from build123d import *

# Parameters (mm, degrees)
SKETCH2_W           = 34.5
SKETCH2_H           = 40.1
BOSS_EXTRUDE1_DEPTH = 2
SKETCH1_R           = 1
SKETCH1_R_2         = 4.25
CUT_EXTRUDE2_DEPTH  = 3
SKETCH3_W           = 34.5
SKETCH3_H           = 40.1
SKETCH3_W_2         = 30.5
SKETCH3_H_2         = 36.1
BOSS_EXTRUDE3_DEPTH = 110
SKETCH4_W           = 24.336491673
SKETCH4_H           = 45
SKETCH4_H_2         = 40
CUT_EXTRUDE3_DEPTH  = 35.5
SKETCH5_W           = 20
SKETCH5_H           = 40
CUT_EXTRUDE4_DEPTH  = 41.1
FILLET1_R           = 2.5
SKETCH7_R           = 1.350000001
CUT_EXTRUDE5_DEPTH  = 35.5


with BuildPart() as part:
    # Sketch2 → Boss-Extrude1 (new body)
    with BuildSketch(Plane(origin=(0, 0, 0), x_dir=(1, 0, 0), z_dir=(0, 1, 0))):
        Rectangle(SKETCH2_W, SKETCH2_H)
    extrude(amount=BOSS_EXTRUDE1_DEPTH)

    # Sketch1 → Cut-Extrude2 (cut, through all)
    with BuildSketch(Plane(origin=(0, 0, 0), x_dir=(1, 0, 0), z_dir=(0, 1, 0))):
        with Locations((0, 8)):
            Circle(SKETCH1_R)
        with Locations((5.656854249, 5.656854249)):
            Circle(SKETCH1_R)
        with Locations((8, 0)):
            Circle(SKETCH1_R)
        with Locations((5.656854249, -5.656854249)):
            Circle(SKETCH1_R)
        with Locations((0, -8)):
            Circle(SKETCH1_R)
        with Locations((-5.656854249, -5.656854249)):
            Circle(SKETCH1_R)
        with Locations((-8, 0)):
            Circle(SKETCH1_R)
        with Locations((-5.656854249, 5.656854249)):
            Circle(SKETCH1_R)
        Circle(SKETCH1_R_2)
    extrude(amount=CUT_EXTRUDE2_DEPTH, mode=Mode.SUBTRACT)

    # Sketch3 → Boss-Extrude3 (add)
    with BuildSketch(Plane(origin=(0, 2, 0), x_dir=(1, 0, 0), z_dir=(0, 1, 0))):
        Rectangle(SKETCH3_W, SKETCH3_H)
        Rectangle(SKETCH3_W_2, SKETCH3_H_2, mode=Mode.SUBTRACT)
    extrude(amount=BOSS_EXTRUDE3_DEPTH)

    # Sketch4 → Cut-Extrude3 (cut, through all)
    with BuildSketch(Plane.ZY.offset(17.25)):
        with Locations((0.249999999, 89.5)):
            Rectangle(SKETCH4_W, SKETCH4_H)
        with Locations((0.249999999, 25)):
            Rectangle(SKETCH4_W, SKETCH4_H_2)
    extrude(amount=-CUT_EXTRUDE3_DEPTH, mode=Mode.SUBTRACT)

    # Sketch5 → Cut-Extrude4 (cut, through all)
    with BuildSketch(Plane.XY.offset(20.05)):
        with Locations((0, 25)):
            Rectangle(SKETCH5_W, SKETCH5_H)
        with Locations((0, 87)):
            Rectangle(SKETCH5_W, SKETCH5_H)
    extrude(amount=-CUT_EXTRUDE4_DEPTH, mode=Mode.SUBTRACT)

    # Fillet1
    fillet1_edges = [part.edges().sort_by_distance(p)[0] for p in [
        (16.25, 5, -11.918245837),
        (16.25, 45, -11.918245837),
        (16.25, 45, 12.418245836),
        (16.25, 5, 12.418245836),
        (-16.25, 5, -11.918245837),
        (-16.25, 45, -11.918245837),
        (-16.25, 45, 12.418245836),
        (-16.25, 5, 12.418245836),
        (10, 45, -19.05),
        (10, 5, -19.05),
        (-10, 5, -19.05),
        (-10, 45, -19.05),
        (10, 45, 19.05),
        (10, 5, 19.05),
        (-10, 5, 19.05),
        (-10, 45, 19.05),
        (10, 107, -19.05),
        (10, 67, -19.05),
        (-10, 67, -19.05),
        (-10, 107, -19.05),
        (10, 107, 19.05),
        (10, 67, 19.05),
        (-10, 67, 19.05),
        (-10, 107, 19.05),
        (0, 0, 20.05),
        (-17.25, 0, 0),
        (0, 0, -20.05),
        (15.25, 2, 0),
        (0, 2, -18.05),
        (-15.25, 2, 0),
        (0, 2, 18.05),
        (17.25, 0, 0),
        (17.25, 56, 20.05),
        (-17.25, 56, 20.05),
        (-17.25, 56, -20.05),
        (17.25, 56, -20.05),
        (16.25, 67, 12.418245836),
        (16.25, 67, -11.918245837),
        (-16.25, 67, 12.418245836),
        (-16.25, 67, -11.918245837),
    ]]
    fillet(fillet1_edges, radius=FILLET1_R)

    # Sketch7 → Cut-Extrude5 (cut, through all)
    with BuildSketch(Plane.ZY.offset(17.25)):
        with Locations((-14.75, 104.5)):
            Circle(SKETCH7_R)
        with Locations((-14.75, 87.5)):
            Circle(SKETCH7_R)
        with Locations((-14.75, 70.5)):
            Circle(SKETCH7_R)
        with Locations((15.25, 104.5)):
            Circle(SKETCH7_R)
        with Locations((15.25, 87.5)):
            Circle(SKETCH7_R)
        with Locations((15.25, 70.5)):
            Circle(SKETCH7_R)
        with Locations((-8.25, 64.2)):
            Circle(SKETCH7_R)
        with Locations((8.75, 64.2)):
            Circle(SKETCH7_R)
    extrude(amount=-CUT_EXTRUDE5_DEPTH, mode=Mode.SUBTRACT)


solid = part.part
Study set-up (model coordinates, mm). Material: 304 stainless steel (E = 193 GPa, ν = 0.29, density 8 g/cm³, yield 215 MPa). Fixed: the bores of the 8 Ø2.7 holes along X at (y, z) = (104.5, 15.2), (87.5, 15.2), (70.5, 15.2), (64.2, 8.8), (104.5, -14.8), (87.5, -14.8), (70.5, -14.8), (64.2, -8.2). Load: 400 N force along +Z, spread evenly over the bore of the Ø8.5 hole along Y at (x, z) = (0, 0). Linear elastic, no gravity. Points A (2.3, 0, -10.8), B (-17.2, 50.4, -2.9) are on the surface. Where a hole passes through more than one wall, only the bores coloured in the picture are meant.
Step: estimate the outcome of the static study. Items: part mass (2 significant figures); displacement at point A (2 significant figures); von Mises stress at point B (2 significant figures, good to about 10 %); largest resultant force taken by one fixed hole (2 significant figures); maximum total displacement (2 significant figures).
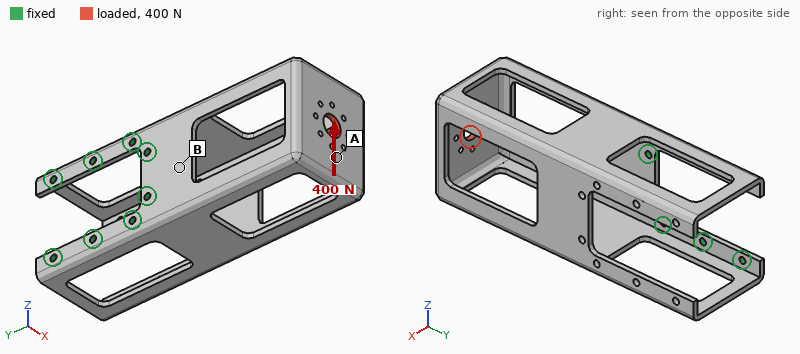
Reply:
150 g
0.13 mm
34 MPa
480 N
0.15 mm
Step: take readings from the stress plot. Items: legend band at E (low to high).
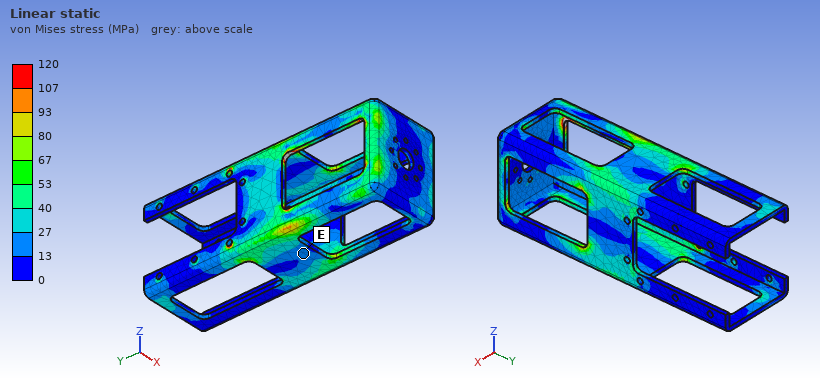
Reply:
13 to 27 MPa
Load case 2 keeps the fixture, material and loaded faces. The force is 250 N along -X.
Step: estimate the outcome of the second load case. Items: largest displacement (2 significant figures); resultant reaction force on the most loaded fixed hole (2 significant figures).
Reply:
0.17 mm
340 N
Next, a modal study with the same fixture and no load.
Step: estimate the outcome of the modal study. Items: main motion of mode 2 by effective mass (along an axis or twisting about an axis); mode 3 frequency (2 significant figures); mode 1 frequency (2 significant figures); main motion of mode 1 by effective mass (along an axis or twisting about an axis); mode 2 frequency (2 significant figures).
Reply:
along X
1600 Hz
790 Hz
along Z
890 Hz
